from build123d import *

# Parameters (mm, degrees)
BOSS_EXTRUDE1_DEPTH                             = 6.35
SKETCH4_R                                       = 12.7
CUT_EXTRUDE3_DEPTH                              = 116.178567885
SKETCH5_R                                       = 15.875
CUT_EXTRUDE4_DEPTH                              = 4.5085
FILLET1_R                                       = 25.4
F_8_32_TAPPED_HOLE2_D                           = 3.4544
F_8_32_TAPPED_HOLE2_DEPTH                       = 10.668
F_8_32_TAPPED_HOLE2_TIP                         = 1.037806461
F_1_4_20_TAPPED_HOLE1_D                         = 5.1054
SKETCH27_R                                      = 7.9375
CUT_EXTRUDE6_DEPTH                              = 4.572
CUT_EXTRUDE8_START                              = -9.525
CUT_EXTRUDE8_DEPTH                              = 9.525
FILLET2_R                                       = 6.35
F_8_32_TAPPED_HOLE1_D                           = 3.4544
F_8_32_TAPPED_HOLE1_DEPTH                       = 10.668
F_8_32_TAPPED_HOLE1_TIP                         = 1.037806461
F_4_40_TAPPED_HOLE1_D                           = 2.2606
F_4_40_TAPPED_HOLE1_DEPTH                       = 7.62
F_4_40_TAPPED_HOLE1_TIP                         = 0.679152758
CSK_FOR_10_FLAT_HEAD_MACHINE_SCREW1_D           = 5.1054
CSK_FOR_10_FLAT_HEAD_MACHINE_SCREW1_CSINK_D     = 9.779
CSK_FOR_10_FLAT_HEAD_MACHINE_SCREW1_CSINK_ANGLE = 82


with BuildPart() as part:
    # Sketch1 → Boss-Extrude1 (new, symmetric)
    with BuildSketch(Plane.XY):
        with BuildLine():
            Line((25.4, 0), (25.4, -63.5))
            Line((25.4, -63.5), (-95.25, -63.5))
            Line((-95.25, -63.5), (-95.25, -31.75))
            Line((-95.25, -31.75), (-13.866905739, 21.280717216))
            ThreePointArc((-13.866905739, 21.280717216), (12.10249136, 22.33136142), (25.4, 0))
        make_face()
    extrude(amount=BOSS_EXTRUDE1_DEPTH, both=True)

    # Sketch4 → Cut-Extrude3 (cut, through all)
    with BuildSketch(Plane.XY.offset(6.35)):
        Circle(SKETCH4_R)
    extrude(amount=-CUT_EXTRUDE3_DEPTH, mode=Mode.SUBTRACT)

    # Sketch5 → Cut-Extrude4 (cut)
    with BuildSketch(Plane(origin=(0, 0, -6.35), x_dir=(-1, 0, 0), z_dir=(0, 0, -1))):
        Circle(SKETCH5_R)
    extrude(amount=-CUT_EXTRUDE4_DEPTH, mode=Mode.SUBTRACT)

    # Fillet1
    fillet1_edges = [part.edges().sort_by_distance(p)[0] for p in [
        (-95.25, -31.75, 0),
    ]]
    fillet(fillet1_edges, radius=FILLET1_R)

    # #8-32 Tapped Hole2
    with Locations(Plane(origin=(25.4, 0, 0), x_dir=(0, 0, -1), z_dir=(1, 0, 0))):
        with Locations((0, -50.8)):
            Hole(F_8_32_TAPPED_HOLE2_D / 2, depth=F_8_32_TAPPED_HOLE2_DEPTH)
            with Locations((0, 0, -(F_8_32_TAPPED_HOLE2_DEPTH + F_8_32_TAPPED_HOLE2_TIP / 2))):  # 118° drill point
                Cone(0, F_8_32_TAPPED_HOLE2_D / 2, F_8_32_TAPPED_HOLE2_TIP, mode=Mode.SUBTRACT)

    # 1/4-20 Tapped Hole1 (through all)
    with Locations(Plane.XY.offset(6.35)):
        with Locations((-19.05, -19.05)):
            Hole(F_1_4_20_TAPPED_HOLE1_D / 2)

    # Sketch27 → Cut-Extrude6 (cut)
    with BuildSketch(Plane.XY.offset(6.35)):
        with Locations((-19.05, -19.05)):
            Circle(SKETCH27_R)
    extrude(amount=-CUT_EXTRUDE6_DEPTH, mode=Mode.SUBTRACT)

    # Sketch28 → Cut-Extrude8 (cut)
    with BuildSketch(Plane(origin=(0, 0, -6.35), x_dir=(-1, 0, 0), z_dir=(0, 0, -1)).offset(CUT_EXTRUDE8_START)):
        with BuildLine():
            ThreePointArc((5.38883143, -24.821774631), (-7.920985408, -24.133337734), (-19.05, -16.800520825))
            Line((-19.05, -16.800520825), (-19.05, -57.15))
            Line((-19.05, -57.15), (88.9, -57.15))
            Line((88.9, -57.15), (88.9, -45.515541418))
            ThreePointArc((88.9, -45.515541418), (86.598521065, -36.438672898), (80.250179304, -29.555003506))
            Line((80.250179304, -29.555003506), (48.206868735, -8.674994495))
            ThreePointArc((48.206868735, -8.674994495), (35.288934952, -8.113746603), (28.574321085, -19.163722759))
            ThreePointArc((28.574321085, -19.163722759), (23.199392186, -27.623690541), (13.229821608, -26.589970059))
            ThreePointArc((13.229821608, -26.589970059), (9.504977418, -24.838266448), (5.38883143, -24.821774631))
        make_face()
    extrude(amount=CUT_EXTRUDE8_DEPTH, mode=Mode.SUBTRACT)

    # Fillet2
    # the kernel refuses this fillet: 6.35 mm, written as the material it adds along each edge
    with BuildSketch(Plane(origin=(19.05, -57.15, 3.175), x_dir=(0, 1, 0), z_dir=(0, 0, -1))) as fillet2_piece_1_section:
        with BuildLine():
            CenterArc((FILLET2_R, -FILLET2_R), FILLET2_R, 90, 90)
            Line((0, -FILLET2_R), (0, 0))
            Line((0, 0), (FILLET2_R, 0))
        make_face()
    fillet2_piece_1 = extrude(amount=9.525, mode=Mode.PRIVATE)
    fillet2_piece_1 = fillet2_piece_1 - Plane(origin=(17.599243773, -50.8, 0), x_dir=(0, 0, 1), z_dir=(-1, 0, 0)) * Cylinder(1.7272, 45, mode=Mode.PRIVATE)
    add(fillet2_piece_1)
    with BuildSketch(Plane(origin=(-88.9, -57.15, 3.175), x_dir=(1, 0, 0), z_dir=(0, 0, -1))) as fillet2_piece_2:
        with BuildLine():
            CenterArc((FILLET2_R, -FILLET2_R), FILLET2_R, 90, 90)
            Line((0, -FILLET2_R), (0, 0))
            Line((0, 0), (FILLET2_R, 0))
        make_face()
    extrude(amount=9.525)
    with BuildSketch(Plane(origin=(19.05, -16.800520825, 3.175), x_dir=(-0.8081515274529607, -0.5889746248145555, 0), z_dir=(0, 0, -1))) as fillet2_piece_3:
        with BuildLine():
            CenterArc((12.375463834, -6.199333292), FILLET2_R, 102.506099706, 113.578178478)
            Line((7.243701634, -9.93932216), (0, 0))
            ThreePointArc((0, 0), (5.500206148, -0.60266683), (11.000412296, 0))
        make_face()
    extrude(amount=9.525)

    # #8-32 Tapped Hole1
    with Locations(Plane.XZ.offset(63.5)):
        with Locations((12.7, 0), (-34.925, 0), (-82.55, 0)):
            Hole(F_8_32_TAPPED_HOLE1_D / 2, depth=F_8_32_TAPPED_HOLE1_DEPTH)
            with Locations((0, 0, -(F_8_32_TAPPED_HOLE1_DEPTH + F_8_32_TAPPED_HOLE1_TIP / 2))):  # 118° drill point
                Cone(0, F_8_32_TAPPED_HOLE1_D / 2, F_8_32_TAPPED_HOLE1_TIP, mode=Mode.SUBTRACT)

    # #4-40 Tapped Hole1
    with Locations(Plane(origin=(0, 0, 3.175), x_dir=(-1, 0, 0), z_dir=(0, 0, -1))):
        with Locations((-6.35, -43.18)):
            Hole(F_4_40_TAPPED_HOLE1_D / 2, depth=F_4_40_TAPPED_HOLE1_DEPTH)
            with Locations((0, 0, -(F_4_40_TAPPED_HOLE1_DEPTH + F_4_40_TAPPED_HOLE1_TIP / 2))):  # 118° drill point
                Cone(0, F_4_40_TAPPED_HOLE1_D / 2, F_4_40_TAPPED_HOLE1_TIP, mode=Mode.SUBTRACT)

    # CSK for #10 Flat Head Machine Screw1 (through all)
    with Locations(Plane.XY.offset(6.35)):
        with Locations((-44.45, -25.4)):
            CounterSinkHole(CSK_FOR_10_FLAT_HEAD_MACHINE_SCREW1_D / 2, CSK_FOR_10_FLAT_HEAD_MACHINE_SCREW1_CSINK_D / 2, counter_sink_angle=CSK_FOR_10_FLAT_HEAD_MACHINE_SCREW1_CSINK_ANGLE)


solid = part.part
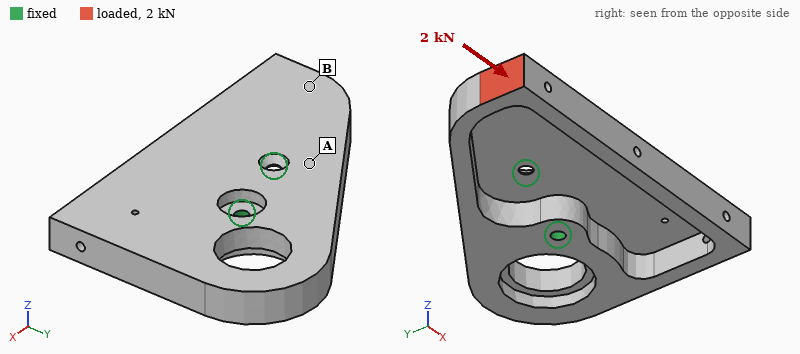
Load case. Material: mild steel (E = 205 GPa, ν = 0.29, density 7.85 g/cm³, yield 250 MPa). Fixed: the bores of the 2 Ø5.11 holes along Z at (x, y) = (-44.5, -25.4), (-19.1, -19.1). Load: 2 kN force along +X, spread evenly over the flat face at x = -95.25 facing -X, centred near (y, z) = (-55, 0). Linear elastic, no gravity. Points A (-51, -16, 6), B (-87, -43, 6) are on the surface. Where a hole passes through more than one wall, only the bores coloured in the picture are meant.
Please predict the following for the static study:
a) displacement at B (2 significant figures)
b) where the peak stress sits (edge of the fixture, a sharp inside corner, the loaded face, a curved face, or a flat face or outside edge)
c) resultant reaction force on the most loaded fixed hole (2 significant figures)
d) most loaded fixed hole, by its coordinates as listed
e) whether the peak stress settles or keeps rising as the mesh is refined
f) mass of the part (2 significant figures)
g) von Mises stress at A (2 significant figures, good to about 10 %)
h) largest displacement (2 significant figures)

32 µm
edge of the fixture
2.4 kN
(-44.5, -25.4)
keeps rising
440 g
26 MPa
47 µm
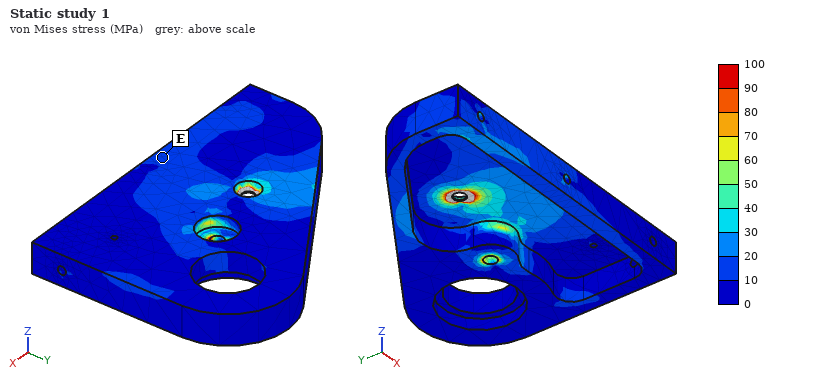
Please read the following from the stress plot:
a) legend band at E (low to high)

10 to 20 MPa
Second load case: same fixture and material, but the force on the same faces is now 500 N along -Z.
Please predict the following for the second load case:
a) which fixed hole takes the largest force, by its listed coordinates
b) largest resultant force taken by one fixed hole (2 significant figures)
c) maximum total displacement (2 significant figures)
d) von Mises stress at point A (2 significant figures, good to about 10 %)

(-44.5, -25.4)
1.1 kN
0.22 mm
82 MPa
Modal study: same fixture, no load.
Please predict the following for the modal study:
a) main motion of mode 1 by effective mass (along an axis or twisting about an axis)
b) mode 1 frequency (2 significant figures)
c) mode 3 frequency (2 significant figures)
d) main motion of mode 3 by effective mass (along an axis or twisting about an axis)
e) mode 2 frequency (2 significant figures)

along Z
1100 Hz
2500 Hz
along Z
1500 Hz
